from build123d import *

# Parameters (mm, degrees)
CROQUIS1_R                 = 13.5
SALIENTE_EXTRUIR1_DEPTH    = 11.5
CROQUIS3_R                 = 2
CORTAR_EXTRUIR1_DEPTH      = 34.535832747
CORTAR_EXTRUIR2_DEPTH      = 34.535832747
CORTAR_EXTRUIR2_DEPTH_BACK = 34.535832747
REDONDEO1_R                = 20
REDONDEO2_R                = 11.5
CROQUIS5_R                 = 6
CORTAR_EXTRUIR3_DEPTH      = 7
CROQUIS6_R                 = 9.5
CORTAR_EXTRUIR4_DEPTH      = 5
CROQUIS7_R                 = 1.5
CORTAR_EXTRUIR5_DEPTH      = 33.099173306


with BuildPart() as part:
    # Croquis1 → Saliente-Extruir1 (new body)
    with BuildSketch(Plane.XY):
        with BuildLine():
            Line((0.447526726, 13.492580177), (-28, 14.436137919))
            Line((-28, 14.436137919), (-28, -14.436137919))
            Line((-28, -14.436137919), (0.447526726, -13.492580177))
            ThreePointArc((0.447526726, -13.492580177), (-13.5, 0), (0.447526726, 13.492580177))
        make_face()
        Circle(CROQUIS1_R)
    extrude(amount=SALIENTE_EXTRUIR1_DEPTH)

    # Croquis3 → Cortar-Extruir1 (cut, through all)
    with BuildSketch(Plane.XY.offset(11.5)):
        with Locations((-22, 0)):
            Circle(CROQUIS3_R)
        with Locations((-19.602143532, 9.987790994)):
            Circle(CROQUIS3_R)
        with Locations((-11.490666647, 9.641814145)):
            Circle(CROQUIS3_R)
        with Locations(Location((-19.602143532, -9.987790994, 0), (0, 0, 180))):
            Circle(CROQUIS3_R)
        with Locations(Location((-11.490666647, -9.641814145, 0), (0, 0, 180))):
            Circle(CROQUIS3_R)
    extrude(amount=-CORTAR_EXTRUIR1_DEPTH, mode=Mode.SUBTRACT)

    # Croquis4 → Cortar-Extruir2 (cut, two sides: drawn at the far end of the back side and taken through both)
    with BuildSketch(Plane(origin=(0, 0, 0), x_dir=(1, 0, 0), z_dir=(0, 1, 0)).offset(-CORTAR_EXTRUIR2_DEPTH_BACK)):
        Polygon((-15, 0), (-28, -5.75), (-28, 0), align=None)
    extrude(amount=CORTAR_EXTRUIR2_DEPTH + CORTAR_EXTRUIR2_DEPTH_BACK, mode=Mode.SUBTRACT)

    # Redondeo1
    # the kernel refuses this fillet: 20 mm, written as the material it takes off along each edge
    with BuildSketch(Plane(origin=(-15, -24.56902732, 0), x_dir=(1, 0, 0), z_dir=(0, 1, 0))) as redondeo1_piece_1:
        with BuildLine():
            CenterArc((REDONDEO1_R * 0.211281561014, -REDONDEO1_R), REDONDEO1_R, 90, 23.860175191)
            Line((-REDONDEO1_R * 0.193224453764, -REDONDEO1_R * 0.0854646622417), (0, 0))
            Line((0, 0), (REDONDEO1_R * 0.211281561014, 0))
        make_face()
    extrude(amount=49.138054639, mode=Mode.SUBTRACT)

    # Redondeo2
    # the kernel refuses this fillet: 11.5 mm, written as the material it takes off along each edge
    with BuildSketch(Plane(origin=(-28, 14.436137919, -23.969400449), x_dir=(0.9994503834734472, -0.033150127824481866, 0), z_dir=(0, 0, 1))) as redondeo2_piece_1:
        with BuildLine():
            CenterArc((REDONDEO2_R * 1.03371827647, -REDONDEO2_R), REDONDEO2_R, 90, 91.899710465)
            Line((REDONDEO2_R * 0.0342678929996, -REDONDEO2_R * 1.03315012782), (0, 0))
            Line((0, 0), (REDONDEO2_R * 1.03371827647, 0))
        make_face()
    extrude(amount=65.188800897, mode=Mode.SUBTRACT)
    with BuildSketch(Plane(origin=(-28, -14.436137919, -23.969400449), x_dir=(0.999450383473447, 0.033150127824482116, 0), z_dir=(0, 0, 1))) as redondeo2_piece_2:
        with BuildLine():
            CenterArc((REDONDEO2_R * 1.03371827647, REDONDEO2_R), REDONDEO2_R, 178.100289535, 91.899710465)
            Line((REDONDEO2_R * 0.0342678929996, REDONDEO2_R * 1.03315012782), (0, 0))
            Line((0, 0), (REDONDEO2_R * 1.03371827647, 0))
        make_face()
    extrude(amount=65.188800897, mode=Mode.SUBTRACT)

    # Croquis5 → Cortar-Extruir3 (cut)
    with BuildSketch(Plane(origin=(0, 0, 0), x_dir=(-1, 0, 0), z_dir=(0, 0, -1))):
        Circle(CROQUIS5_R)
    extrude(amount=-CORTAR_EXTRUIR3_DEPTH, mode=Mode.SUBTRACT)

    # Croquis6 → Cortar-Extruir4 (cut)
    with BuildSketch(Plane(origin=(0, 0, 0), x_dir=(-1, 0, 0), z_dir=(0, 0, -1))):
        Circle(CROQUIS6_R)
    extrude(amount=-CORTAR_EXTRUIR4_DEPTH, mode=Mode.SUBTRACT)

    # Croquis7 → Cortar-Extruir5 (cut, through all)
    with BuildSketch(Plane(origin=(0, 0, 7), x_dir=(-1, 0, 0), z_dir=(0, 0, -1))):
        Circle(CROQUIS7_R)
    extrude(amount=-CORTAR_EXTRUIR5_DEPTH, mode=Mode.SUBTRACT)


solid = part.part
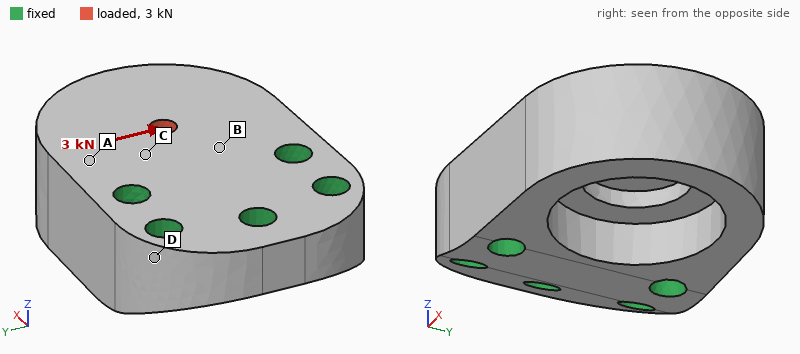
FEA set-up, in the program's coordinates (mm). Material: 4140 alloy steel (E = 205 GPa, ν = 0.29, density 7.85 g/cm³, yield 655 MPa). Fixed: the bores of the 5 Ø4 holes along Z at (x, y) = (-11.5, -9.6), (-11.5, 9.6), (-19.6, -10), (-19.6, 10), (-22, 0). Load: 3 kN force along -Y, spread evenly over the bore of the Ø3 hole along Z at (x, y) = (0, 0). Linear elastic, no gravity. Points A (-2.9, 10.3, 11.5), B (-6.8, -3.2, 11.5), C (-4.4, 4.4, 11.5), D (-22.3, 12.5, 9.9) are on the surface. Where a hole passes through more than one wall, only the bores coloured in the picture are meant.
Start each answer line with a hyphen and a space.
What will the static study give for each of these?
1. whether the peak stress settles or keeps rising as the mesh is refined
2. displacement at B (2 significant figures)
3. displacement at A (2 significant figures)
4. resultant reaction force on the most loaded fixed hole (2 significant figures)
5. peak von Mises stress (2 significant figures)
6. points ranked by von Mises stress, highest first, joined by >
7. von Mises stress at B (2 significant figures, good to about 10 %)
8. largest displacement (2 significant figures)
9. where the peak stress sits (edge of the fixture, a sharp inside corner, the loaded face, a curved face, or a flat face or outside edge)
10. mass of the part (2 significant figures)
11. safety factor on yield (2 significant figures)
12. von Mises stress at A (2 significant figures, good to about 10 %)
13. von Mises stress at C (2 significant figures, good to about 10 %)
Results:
- settles
- 1.1 µm
- 2.2 µm
- 2.0 kN
- 130 MPa
- C > B > A > D
- 34 MPa
- 4.6 µm
- the loaded face
- 66 g
- 5.0
- 23 MPa
- 44 MPa
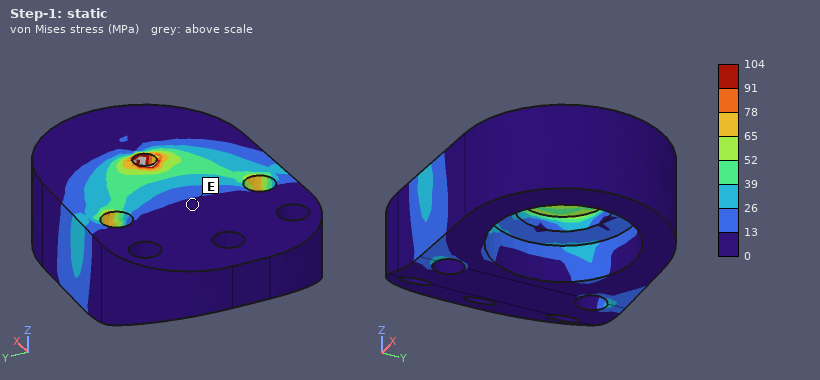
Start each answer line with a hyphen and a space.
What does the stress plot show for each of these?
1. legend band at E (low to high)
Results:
- 0 to 13 MPa
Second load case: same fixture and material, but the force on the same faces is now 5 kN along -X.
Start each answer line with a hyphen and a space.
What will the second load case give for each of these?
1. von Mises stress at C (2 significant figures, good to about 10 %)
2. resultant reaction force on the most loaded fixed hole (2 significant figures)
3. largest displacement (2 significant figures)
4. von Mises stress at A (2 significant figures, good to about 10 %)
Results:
- 52 MPa
- 1.9 kN
- 6.5 µm
- 28 MPa
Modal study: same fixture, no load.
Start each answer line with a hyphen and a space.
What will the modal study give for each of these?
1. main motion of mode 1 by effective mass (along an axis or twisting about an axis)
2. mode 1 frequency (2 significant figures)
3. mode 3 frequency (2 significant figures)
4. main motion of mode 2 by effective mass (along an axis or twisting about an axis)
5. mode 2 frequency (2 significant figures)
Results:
- along Z
- 14 kHz
- 30 kHz
- along Y
- 21 kHz
